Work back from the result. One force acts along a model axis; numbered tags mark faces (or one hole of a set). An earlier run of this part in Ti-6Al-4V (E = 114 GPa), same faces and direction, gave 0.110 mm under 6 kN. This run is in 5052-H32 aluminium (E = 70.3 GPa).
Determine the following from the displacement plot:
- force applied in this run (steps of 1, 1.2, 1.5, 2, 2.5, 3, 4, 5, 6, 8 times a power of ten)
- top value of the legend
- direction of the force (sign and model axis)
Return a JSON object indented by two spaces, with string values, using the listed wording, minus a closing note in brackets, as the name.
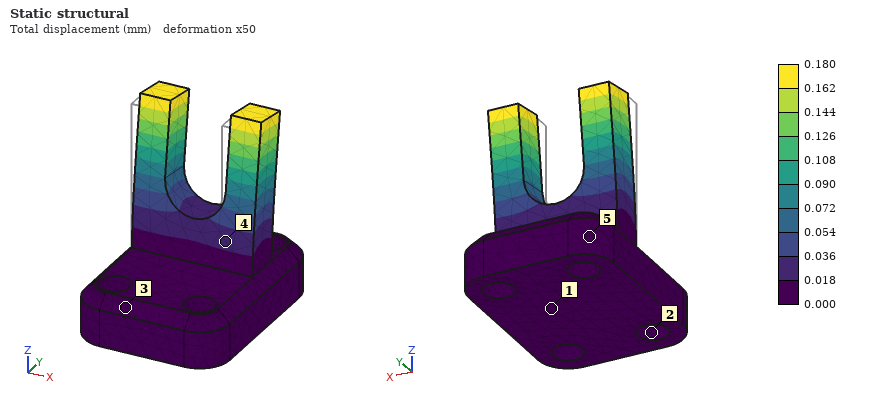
{
  "force applied in this run": "6 kN",
  "top value of the legend": "0.180 mm",
  "direction of the force": "+Y"
}
